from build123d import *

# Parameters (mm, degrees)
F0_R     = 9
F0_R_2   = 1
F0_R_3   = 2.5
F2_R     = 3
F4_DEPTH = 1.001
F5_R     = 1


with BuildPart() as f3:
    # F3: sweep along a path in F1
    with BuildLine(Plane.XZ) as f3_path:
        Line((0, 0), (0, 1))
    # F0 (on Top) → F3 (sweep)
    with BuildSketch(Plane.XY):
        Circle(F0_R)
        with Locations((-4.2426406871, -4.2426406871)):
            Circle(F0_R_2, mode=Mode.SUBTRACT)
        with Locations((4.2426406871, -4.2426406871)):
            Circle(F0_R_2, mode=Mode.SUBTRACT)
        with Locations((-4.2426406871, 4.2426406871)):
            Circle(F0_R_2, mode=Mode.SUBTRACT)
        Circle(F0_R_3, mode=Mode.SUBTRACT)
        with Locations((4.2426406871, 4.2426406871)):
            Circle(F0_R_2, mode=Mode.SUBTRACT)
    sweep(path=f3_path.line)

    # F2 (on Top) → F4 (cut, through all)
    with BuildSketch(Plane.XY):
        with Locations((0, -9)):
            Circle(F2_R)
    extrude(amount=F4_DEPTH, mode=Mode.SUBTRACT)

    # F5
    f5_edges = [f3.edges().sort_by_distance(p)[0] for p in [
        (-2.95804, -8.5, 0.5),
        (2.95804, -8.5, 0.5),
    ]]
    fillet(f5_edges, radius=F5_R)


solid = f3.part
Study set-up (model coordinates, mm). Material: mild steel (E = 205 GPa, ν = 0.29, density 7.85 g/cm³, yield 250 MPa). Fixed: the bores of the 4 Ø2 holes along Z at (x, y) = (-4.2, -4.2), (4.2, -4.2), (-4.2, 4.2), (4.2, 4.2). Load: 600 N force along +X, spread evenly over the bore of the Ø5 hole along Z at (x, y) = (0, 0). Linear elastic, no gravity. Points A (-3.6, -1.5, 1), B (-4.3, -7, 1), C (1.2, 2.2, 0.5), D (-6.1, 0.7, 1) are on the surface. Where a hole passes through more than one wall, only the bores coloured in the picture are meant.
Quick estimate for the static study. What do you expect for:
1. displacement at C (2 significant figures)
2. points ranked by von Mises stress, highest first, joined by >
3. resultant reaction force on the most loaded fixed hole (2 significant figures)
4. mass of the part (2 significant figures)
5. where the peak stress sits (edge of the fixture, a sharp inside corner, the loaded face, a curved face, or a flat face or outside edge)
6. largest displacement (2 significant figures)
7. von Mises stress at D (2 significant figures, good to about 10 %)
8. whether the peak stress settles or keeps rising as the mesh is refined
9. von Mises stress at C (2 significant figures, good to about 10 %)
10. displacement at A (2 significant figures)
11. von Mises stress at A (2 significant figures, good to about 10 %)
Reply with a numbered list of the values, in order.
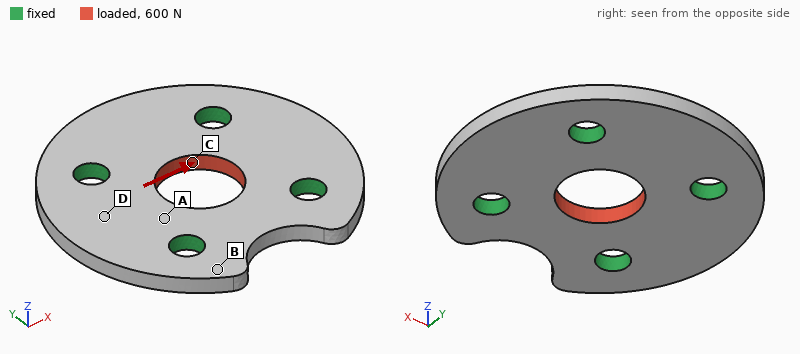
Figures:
1. 0.71 µm
2. C > A > D > B
3. 150 N
4. 1.6 g
5. edge of the fixture
6. 0.94 µm
7. 15 MPa
8. keeps rising
9. 63 MPa
10. 0.59 µm
11. 30 MPa
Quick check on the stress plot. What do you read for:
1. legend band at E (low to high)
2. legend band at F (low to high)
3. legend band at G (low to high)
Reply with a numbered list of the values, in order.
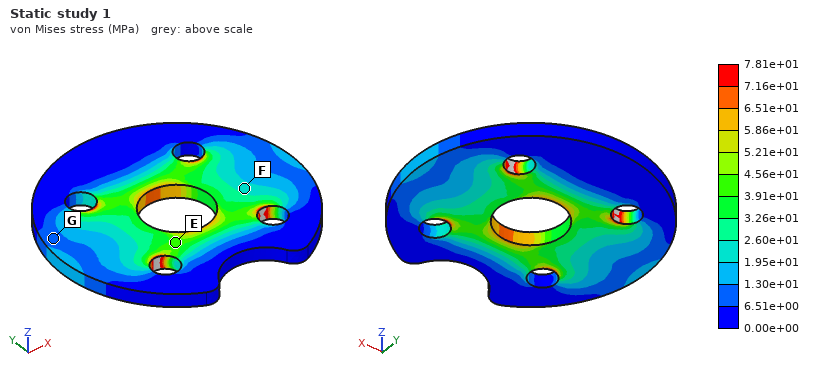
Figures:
1. 3.91e+01 to 4.56e+01 MPa
2. 1.95e+01 to 2.60e+01 MPa
3. 6.51e+00 to 1.30e+01 MPa
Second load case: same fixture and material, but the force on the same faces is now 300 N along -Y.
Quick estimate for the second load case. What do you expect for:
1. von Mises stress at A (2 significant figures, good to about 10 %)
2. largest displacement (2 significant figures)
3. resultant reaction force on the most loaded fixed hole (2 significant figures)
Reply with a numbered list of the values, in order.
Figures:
1. 17 MPa
2. 0.56 µm
3. 80 N
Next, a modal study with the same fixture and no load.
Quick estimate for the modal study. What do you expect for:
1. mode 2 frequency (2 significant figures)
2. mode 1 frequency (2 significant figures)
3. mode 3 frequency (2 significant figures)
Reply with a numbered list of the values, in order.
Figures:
1. 46 kHz
2. 45 kHz
3. 46 kHz
